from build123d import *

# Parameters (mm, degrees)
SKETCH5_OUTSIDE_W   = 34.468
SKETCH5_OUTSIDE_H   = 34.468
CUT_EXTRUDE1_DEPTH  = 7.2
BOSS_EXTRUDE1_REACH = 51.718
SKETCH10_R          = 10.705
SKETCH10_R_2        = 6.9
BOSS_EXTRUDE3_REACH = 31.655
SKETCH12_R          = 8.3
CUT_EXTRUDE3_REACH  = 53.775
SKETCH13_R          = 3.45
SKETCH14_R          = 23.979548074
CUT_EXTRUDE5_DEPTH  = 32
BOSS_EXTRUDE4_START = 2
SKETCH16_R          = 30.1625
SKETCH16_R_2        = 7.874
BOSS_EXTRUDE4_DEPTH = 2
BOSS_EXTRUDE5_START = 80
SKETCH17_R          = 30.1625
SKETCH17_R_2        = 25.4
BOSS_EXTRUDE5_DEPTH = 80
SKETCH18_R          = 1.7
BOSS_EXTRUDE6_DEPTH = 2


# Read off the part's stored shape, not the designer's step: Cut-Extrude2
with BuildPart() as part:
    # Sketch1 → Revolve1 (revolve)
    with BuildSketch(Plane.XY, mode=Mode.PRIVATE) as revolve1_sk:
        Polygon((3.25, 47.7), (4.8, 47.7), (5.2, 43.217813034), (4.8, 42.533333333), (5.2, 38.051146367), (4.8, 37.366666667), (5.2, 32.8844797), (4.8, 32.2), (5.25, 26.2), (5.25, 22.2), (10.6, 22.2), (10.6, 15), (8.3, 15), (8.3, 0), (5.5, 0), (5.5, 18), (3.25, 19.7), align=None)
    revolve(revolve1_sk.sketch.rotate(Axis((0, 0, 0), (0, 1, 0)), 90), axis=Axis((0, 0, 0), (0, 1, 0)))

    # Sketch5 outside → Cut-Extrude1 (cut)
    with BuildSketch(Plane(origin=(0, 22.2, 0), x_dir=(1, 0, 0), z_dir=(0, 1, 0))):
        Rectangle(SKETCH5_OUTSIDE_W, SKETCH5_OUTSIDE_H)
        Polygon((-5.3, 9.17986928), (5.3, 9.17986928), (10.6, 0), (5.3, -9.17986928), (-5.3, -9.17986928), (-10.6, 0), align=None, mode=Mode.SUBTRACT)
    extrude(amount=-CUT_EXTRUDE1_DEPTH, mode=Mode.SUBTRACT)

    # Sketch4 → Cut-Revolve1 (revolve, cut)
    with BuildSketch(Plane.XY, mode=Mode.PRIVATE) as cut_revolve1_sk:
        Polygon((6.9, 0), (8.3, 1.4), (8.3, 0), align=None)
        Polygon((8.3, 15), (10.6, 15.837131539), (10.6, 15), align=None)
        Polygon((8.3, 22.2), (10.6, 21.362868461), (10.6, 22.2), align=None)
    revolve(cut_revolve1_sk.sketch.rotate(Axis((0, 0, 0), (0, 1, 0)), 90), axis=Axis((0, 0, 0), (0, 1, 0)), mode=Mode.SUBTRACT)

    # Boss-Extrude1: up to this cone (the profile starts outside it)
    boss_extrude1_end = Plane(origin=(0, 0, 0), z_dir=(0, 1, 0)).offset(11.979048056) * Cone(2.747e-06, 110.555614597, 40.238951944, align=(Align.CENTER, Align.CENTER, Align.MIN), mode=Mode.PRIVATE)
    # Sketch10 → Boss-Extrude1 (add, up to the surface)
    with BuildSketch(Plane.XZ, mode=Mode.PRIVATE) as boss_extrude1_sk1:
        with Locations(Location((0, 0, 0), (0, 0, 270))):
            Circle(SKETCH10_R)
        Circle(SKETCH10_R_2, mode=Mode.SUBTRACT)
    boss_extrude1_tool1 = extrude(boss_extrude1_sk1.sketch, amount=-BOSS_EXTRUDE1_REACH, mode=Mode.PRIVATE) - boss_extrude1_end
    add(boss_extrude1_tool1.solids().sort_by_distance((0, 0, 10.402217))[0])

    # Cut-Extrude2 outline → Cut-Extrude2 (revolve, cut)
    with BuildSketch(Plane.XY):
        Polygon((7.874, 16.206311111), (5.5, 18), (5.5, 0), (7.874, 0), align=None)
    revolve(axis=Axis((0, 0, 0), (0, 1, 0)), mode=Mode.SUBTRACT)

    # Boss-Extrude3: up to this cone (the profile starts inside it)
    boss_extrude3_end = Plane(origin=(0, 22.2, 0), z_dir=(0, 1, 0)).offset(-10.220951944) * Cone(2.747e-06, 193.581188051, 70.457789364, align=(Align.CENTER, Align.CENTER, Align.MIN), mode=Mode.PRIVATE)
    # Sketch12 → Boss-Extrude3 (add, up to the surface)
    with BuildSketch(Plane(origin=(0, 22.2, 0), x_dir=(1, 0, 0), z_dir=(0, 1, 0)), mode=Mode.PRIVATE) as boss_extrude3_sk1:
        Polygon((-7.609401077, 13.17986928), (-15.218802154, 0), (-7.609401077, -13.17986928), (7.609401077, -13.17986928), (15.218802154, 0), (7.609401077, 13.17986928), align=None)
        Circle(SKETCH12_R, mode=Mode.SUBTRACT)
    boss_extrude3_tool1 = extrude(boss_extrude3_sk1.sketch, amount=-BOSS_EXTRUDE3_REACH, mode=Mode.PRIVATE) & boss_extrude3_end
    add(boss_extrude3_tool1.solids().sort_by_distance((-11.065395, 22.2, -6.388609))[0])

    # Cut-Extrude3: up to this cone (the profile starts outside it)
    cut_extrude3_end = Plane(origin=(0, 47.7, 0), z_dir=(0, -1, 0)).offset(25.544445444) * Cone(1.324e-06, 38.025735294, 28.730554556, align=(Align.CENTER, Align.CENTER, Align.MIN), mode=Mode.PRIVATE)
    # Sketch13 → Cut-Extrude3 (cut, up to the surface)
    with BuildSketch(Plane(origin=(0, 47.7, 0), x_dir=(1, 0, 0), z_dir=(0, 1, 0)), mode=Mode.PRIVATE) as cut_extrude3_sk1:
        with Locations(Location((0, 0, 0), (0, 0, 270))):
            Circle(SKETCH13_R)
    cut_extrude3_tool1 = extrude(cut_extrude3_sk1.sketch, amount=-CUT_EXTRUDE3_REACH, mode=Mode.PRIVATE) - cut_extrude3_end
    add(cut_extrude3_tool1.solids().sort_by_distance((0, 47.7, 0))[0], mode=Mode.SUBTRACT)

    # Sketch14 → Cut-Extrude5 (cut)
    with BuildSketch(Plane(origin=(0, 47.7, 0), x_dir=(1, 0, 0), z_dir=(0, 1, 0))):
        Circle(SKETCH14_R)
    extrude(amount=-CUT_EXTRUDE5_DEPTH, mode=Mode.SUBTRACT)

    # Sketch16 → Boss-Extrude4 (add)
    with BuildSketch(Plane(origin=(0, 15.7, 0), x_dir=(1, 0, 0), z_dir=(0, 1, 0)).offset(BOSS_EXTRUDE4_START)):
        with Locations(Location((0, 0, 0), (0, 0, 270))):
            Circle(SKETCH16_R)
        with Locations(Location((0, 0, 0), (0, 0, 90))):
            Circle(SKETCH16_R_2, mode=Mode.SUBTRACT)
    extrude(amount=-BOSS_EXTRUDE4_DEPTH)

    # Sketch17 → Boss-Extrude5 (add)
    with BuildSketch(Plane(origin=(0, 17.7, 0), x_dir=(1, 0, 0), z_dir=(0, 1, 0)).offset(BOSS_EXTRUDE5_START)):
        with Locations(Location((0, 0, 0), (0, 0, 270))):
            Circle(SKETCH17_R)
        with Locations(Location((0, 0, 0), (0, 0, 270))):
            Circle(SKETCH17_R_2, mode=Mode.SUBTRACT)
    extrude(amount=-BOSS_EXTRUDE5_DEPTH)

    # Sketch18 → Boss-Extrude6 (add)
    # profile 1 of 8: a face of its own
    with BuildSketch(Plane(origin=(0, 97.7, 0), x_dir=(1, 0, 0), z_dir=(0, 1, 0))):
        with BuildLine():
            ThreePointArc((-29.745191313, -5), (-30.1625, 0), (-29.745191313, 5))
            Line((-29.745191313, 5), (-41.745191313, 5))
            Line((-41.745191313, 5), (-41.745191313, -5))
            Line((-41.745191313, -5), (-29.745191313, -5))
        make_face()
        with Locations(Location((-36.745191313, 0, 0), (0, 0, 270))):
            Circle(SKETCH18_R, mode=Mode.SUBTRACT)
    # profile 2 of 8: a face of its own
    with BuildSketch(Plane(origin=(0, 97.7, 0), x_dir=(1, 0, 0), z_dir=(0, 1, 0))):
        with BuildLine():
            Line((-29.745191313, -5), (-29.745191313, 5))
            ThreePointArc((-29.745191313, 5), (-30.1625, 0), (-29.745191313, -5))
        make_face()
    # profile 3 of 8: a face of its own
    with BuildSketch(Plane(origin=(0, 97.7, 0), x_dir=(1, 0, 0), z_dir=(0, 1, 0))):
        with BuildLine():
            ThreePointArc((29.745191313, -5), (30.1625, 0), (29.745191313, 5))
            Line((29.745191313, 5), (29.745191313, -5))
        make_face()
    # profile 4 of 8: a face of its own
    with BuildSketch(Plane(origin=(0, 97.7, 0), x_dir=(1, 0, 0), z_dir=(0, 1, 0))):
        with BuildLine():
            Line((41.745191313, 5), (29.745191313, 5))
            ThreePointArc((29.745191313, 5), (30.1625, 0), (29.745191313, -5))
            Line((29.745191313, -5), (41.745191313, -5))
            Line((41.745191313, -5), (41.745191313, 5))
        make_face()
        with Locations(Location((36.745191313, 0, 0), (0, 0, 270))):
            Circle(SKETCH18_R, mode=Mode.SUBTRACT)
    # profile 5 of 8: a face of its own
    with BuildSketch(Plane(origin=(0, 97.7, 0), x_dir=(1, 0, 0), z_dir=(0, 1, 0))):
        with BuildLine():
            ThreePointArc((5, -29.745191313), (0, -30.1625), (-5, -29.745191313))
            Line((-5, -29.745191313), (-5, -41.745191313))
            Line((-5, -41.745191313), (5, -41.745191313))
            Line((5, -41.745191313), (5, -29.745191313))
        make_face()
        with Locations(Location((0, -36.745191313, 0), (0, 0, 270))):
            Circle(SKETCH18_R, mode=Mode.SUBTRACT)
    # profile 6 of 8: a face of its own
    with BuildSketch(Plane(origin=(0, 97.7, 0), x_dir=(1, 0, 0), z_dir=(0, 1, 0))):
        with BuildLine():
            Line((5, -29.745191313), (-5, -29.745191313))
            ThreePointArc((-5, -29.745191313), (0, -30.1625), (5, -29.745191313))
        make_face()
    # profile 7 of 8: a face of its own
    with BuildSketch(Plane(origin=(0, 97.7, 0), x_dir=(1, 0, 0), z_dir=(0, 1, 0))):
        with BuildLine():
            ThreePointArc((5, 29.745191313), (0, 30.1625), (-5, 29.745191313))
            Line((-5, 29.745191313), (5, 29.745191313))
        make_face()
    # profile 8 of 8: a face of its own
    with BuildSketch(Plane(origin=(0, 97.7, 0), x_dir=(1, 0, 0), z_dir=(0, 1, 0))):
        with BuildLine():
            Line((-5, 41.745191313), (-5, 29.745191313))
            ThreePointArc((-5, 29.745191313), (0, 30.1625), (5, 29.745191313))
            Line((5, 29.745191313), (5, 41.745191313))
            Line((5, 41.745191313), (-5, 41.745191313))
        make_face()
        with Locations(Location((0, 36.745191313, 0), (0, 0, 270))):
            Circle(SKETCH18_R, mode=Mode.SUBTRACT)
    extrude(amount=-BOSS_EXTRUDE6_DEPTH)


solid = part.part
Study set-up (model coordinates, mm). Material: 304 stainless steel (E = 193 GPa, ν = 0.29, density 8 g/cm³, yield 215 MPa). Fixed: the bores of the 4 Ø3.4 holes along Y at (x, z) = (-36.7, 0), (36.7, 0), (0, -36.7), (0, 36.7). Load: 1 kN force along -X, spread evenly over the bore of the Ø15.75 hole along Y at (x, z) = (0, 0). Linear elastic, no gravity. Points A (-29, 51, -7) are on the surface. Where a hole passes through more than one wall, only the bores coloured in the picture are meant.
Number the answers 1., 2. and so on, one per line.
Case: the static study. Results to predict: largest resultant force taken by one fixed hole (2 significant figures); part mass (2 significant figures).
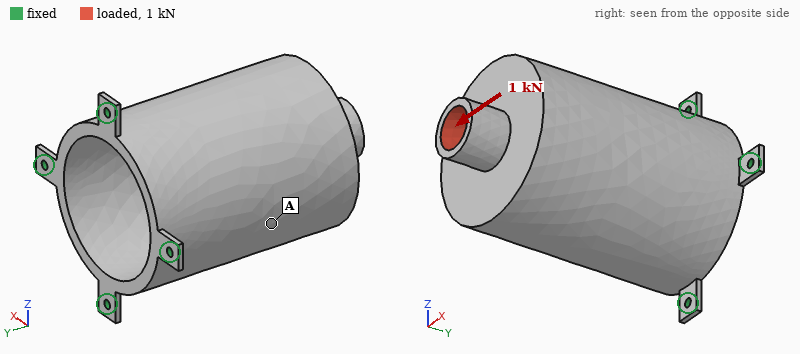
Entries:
1. 1.4 kN
2. 600 g
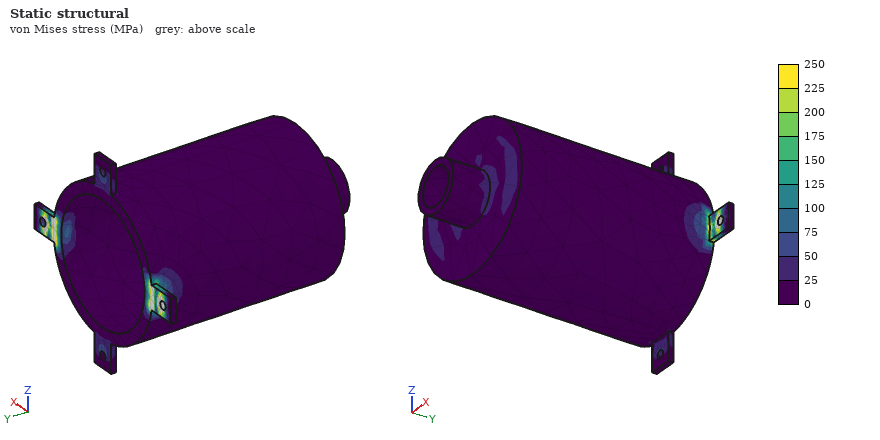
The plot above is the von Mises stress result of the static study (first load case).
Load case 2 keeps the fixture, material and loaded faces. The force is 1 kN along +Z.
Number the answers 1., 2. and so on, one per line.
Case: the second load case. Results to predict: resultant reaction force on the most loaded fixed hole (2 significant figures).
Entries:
1. 1.4 kN
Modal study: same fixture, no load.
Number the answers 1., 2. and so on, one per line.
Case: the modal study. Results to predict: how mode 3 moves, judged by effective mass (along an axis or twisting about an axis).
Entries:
1. along Y
